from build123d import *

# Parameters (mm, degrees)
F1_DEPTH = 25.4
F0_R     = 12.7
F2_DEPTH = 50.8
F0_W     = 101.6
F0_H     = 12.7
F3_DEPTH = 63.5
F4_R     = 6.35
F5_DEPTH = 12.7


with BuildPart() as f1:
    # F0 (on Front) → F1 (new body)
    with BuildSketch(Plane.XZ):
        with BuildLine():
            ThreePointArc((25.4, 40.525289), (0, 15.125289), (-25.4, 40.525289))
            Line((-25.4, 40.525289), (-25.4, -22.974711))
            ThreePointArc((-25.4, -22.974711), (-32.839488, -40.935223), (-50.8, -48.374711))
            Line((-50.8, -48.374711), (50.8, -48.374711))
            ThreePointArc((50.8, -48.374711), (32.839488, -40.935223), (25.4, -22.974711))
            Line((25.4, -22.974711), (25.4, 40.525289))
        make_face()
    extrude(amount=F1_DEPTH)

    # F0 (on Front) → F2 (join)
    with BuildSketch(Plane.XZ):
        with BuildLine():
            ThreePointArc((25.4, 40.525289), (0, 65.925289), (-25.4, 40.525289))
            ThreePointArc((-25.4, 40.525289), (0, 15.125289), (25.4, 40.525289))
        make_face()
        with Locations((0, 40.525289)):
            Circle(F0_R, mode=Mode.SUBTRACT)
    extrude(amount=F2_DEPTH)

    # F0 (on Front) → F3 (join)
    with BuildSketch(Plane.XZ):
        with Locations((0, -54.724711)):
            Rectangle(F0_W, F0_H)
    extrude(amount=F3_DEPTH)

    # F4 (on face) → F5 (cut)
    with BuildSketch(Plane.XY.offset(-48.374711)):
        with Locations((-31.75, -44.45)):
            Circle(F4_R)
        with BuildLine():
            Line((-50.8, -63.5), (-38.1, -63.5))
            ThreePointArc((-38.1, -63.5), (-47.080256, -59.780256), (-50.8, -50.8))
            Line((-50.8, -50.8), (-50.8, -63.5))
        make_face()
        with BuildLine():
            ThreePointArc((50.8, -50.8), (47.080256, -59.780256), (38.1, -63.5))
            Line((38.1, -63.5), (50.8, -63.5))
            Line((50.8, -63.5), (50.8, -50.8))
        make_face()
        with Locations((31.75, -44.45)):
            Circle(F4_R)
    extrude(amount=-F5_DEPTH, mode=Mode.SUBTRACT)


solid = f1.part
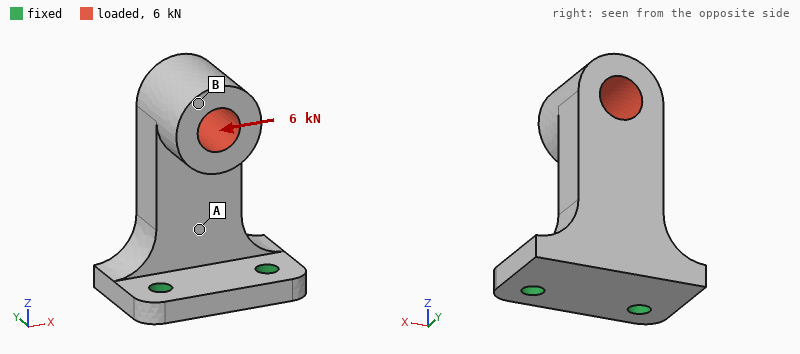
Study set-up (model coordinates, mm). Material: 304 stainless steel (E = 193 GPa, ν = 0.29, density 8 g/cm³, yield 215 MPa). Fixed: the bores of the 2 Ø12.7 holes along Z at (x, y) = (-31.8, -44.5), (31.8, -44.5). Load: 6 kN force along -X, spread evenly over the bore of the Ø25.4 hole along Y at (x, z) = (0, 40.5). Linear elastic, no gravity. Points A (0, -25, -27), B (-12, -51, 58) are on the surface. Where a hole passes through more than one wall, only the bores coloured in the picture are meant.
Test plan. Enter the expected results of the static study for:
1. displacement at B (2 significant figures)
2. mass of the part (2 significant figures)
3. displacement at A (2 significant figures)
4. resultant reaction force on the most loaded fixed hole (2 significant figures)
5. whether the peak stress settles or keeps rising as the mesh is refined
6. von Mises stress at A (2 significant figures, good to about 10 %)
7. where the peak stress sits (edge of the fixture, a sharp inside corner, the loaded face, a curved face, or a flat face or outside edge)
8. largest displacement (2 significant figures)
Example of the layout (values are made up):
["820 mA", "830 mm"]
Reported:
["0.13 mm", "2.0 kg", "0.023 mm", "9.1 kN", "keeps rising", "30 MPa", "edge of the fixture", "0.14 mm"]
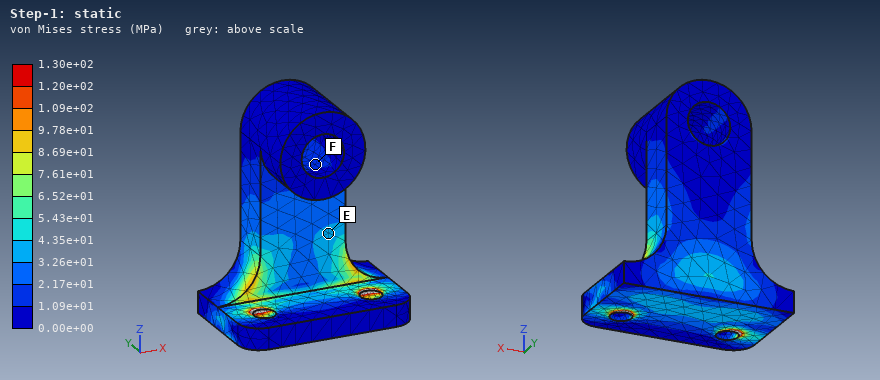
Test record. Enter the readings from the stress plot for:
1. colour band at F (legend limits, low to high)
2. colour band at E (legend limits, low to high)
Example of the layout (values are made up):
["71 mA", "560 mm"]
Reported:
["1.09e+01 to 2.17e+01 MPa", "3.26e+01 to 4.35e+01 MPa"]
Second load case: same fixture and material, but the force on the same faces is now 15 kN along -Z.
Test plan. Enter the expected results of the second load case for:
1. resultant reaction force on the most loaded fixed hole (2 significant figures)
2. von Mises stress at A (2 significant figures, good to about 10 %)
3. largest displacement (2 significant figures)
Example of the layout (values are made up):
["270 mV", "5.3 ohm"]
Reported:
["7.6 kN", "36 MPa", "52 µm"]
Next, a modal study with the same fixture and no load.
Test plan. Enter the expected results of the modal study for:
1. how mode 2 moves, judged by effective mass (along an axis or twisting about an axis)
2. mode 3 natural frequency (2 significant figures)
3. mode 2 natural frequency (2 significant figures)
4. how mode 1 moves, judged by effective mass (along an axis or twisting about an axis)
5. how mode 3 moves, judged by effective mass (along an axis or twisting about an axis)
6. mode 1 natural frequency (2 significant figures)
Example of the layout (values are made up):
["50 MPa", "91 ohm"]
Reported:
["along X", "2900 Hz", "1400 Hz", "along Y", "along Z", "600 Hz"]
